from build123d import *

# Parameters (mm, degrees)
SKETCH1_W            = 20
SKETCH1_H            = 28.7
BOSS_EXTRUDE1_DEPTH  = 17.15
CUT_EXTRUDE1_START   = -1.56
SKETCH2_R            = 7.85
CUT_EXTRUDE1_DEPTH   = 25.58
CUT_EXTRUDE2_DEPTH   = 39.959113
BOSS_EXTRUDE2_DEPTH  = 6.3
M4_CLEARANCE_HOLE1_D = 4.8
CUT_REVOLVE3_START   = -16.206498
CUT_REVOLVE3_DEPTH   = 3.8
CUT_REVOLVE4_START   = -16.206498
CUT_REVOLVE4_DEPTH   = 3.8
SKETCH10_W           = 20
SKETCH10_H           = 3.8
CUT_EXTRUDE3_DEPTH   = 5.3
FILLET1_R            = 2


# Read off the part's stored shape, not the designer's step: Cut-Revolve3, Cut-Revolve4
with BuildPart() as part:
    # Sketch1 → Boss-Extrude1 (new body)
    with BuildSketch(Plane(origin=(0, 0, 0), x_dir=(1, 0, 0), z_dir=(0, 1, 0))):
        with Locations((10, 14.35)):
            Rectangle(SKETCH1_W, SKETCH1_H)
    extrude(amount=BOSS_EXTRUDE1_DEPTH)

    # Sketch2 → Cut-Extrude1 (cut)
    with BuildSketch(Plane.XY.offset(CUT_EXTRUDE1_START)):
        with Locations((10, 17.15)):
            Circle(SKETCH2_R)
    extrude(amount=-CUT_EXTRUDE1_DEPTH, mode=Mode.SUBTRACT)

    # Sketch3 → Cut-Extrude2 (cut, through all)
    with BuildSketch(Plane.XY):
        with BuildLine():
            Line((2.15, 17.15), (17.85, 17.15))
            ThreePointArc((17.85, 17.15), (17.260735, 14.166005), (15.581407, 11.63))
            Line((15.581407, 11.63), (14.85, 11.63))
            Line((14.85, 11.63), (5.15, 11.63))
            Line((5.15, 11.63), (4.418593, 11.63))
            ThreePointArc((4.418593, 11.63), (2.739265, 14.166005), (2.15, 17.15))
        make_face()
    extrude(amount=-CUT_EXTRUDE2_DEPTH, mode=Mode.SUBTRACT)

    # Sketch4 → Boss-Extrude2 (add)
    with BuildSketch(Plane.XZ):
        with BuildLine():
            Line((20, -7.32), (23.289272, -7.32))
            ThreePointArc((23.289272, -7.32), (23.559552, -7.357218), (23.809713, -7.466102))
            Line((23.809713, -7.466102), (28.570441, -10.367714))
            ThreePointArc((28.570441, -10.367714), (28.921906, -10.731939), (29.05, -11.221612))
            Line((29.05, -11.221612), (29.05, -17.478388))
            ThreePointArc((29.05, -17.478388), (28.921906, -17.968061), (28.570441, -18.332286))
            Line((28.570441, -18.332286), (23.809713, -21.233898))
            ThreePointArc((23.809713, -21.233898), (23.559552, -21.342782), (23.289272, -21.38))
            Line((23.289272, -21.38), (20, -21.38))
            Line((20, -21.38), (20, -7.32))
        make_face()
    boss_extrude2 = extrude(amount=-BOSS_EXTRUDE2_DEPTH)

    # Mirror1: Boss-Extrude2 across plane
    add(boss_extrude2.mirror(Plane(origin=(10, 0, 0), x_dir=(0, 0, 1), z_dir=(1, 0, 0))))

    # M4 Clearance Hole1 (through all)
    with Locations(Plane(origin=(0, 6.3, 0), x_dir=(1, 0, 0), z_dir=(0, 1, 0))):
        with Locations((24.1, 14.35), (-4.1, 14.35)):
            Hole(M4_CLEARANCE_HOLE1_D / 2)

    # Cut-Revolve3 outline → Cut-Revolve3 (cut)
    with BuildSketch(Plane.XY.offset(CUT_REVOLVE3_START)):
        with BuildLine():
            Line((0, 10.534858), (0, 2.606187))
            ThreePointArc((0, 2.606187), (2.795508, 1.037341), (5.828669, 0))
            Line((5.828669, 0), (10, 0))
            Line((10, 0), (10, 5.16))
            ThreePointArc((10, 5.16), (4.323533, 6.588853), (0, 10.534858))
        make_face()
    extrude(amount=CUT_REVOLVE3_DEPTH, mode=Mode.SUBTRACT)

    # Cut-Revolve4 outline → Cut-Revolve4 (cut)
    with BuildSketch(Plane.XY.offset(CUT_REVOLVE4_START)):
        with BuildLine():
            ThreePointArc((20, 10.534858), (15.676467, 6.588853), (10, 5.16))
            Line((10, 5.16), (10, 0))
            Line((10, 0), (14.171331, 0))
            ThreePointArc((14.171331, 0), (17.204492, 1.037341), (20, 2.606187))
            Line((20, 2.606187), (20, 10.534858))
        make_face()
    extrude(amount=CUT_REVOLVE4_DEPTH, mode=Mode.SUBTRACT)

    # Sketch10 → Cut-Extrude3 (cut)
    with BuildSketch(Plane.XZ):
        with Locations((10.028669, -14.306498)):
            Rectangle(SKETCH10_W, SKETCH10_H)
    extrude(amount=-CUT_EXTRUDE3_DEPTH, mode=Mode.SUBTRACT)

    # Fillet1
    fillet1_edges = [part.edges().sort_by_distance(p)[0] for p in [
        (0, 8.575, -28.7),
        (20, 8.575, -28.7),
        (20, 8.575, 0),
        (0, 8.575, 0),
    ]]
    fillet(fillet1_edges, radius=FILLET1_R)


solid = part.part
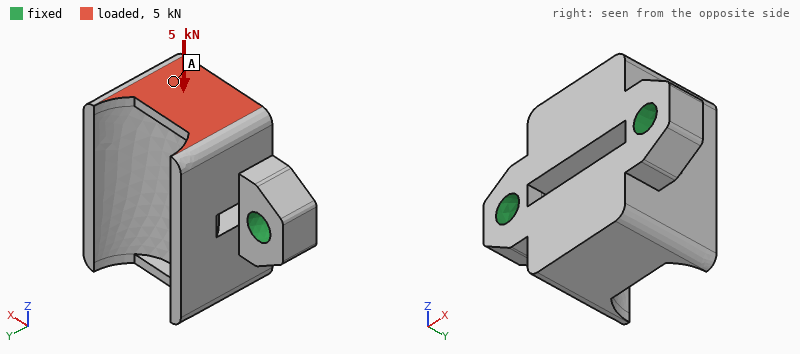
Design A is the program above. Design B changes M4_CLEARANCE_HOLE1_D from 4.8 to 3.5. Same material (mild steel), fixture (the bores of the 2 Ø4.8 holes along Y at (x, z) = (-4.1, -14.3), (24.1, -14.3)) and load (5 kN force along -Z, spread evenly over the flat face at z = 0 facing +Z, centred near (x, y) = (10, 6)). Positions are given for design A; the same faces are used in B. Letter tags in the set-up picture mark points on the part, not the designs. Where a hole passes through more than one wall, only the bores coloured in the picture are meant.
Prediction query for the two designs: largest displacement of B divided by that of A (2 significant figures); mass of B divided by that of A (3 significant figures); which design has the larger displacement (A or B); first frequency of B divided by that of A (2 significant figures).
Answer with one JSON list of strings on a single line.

["1.1", "1.01", "B", "0.90"]
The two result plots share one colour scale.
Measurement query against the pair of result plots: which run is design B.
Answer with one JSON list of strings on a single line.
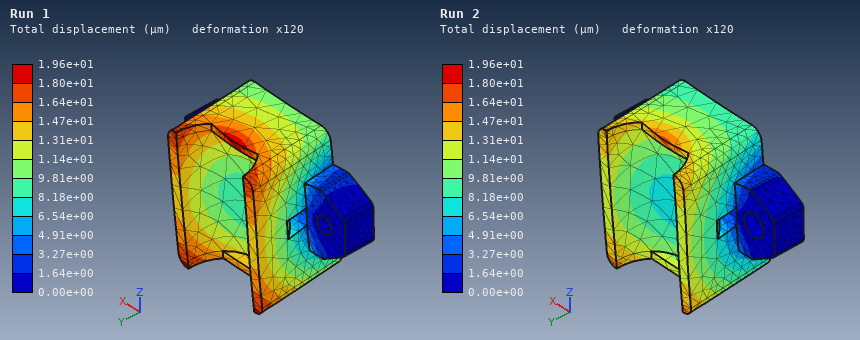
["Run 1"]
